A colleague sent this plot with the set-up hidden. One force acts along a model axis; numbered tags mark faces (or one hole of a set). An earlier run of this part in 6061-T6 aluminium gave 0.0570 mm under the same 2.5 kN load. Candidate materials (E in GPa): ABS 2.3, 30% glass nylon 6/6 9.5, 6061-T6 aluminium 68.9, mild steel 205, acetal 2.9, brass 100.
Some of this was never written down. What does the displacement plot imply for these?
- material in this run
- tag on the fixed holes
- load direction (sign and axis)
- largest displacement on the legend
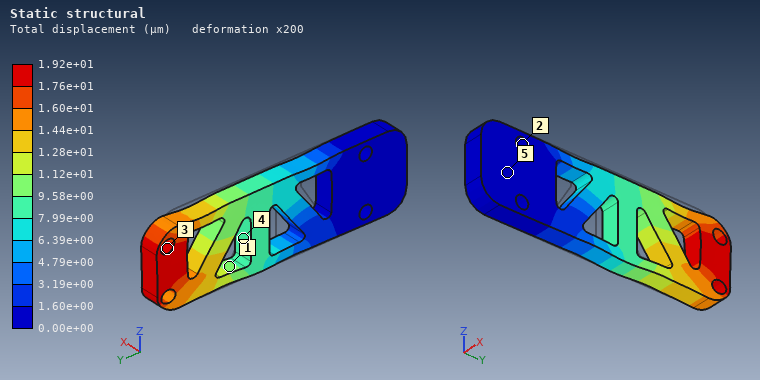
mild steel
2
+Y
1.92e+01 µm
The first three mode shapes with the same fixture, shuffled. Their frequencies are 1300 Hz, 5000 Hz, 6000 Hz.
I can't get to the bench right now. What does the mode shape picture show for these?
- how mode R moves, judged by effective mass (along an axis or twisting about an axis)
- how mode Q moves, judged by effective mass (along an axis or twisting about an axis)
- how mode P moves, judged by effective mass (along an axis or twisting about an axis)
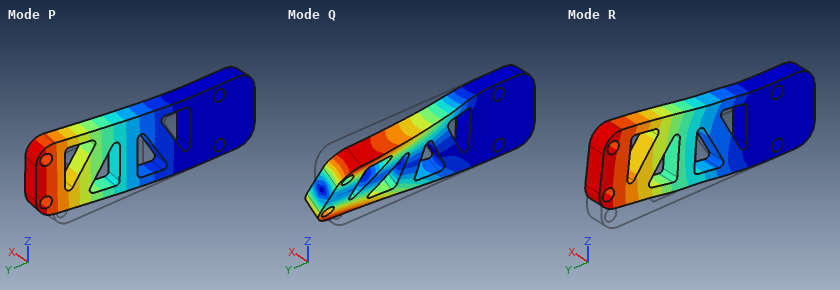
along Z
twisting about Y
along X
